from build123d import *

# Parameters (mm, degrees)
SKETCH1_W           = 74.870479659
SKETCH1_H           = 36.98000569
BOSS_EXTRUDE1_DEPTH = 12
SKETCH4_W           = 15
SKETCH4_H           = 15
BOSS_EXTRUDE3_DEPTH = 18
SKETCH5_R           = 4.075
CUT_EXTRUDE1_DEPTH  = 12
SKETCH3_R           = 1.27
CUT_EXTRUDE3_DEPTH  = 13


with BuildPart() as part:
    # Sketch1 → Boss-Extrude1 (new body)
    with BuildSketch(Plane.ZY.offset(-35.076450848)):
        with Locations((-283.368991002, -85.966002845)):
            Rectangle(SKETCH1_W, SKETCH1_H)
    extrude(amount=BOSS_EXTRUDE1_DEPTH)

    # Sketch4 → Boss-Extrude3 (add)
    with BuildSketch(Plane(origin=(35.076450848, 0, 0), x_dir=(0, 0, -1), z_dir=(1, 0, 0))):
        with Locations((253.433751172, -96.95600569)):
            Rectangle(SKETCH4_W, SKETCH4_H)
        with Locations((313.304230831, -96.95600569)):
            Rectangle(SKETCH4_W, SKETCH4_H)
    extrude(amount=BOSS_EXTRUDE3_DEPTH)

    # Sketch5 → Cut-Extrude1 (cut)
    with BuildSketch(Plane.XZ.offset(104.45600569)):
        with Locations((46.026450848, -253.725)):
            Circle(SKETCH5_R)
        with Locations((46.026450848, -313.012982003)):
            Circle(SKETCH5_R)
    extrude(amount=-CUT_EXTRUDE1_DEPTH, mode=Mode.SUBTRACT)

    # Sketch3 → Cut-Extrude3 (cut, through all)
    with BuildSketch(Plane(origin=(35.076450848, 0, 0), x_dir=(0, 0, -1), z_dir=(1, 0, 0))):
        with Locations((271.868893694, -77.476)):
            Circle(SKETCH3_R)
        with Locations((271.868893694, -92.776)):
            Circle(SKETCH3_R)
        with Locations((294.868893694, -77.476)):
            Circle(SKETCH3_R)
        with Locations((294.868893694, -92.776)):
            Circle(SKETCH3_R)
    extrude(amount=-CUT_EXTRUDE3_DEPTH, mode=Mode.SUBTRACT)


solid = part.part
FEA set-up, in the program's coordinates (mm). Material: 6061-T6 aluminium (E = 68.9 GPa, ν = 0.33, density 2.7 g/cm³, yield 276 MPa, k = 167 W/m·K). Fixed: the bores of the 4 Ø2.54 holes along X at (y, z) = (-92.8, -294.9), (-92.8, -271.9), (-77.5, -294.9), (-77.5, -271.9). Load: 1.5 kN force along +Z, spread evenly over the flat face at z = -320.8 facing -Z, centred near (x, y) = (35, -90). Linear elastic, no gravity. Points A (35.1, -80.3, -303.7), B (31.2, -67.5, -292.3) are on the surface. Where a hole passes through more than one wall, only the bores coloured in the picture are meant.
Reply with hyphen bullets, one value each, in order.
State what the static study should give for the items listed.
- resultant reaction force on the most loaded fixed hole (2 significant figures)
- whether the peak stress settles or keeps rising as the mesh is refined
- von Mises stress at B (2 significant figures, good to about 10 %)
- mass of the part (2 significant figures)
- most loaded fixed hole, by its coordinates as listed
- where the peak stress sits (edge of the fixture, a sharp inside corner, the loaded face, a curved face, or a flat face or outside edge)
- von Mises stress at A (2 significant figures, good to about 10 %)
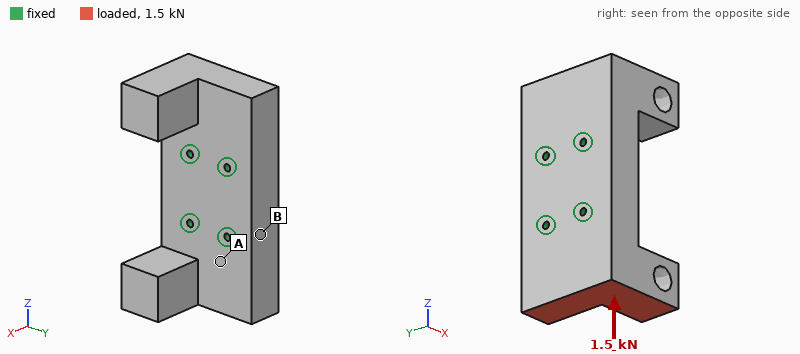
- 870 N
- keeps rising
- 2.9 MPa
- 110 g
- (-92.8, -294.9)
- edge of the fixture
- 9.7 MPa
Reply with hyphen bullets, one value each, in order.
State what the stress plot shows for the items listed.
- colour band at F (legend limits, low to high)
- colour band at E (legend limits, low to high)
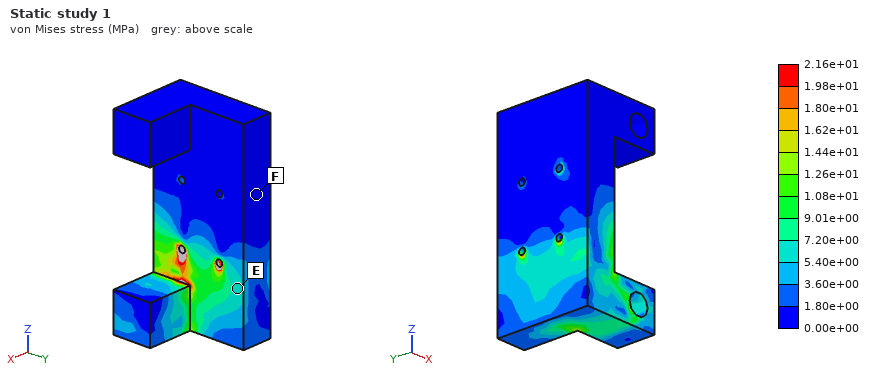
- 0.00e+00 to 1.80e+00 MPa
- 5.40e+00 to 7.20e+00 MPa
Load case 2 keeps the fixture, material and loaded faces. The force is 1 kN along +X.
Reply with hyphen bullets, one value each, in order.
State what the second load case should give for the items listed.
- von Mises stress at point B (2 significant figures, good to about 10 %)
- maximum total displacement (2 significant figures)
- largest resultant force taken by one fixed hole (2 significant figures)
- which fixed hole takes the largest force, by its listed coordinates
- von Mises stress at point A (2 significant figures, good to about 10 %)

- 7.1 MPa
- 39 µm
- 890 N
- (-92.8, -294.9)
- 18 MPa
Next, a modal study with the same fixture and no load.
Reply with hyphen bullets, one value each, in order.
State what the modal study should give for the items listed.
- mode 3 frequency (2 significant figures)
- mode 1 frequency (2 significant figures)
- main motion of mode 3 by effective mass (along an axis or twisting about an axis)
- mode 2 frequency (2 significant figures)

- 10 kHz
- 7400 Hz
- twisting about X
- 7500 Hz
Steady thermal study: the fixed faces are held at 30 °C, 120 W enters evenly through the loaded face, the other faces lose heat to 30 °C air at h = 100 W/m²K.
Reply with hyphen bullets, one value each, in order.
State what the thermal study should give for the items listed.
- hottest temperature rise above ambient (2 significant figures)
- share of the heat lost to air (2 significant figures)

- 54 K
- 9.3 %
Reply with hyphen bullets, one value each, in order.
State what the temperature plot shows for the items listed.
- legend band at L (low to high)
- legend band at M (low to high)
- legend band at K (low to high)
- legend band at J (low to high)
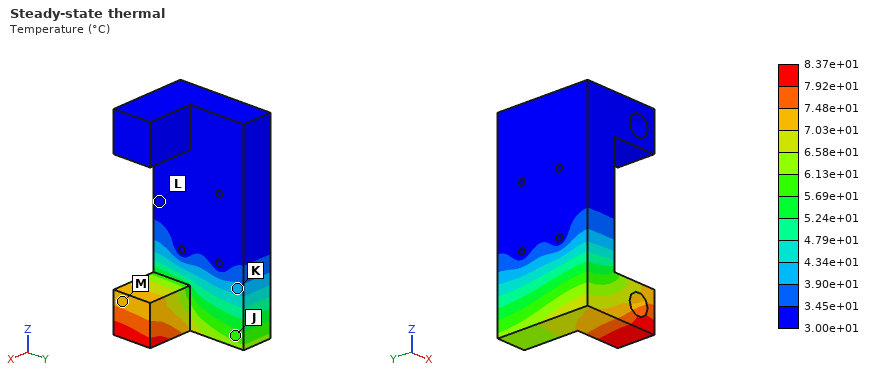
- 3.00e+01 to 3.45e+01 °C
- 7.03e+01 to 7.48e+01 °C
- 3.90e+01 to 4.34e+01 °C
- 5.69e+01 to 6.13e+01 °C
